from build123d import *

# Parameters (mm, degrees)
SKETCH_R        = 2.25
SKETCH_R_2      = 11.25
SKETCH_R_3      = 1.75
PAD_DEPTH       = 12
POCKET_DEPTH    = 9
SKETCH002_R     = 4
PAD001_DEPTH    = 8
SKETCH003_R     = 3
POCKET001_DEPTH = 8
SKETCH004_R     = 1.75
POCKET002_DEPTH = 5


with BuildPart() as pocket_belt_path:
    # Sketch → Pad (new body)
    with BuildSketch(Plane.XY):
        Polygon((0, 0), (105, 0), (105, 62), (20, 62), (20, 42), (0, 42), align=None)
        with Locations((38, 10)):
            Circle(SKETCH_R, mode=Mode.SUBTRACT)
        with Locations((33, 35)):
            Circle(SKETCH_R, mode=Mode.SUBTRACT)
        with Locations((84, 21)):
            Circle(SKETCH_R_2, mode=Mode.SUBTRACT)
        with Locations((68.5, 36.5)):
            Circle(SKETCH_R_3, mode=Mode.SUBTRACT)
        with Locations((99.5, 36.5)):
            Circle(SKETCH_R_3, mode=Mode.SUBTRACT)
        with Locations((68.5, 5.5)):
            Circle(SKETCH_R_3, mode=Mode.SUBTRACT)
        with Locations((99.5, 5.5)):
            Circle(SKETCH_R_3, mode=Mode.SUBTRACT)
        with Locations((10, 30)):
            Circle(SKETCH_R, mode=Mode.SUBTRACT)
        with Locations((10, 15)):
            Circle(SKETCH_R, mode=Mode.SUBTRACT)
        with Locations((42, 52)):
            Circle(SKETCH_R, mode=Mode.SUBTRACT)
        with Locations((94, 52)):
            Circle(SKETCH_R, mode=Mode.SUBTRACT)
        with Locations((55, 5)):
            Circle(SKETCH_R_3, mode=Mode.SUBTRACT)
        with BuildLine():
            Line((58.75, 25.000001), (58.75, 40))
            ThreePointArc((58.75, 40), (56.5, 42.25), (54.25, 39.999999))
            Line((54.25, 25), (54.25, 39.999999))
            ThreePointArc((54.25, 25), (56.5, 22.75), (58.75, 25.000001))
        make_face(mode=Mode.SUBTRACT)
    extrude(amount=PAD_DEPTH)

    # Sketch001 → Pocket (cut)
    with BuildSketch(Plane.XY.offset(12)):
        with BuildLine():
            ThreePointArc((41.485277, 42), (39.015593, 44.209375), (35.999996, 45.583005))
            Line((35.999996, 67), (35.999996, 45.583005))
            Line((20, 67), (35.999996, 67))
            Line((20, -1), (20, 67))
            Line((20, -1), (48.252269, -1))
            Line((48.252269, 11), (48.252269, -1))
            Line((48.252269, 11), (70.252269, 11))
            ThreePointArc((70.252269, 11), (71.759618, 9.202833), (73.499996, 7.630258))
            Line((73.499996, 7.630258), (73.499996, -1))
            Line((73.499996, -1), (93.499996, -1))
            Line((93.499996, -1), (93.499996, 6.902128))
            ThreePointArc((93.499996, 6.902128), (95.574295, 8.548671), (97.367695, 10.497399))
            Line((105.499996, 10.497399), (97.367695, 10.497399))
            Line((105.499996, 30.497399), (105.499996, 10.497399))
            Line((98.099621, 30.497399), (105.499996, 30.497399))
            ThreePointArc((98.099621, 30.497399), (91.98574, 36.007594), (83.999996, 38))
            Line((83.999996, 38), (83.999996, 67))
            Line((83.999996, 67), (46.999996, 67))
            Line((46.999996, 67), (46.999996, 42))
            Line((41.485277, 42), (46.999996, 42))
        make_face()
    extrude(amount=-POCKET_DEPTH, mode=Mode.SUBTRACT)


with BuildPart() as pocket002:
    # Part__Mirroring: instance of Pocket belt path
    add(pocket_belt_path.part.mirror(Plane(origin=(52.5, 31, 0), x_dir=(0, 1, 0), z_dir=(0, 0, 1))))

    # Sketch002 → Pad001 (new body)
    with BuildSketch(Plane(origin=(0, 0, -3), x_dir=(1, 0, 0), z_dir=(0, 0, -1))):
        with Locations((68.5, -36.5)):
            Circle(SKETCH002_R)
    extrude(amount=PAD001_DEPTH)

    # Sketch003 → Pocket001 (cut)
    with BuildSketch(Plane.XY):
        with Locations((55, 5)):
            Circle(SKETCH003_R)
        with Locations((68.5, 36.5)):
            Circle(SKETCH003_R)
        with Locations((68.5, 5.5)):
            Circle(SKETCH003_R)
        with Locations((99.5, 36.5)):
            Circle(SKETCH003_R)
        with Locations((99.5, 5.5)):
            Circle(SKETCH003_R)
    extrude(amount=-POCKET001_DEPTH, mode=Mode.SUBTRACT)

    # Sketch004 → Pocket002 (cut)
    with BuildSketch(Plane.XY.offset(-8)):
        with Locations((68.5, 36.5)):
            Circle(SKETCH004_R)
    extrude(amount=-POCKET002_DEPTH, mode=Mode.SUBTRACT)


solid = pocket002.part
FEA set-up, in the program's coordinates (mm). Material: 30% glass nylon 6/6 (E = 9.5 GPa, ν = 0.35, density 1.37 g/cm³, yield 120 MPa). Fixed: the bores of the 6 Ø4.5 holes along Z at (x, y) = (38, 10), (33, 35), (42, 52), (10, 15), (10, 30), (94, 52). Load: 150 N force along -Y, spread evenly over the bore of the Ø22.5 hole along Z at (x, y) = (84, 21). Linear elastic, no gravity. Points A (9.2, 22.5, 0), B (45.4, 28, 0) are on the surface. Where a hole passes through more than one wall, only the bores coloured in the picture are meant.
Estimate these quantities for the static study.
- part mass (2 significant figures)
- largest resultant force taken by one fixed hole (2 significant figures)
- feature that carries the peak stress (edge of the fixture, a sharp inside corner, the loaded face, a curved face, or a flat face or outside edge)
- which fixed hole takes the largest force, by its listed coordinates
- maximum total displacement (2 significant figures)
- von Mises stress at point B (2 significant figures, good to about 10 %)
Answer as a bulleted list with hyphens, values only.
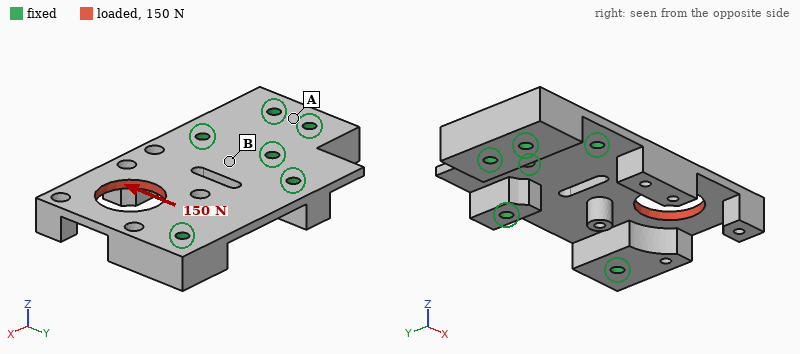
- 46 g
- 110 N
- a curved face
- (94, 52)
- 15 µm
- 0.71 MPa
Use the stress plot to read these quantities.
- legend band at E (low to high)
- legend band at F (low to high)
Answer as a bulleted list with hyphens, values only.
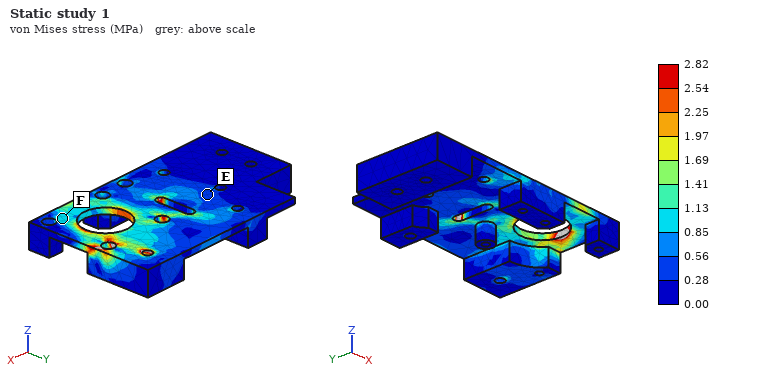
- 0.28 to 0.56 MPa
- 0.85 to 1.13 MPa
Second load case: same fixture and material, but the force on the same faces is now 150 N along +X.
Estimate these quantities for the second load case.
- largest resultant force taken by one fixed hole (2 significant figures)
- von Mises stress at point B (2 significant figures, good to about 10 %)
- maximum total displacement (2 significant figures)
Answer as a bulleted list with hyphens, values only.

- 56 N
- 0.41 MPa
- 10 µm
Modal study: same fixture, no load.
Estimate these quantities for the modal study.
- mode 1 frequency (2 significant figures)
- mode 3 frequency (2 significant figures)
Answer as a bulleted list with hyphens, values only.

- 870 Hz
- 3200 Hz
